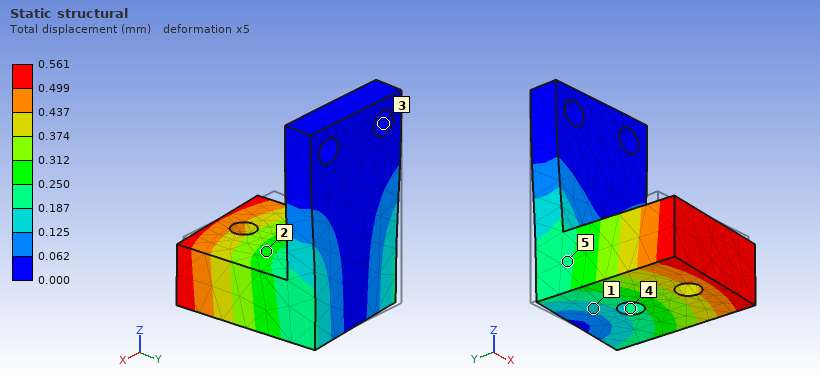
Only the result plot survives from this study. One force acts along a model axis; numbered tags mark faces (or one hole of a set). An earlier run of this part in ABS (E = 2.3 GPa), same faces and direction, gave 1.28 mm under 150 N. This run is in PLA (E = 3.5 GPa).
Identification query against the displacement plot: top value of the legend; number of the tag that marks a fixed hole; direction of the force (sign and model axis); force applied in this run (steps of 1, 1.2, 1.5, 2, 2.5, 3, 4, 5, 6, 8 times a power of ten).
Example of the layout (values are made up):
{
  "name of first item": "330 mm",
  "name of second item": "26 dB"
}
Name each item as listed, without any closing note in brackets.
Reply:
{
  "top value of the legend": "0.561 mm",
  "number of the tag that marks a fixed hole": "3",
  "direction of the force": "+X",
  "force applied in this run": "100 N"
}
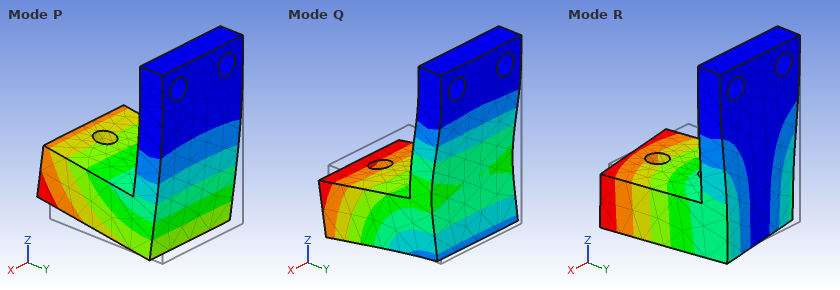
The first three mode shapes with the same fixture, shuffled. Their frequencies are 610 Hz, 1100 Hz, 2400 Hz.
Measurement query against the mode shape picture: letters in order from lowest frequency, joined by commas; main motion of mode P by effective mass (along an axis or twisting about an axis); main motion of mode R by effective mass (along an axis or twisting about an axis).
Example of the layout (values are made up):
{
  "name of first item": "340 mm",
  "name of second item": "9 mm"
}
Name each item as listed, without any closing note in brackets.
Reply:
{
  "letters in order from lowest frequency, joined by commas": "P, R, Q",
  "main motion of mode P by effective mass": "along Y",
  "main motion of mode R by effective mass": "along X"
}
